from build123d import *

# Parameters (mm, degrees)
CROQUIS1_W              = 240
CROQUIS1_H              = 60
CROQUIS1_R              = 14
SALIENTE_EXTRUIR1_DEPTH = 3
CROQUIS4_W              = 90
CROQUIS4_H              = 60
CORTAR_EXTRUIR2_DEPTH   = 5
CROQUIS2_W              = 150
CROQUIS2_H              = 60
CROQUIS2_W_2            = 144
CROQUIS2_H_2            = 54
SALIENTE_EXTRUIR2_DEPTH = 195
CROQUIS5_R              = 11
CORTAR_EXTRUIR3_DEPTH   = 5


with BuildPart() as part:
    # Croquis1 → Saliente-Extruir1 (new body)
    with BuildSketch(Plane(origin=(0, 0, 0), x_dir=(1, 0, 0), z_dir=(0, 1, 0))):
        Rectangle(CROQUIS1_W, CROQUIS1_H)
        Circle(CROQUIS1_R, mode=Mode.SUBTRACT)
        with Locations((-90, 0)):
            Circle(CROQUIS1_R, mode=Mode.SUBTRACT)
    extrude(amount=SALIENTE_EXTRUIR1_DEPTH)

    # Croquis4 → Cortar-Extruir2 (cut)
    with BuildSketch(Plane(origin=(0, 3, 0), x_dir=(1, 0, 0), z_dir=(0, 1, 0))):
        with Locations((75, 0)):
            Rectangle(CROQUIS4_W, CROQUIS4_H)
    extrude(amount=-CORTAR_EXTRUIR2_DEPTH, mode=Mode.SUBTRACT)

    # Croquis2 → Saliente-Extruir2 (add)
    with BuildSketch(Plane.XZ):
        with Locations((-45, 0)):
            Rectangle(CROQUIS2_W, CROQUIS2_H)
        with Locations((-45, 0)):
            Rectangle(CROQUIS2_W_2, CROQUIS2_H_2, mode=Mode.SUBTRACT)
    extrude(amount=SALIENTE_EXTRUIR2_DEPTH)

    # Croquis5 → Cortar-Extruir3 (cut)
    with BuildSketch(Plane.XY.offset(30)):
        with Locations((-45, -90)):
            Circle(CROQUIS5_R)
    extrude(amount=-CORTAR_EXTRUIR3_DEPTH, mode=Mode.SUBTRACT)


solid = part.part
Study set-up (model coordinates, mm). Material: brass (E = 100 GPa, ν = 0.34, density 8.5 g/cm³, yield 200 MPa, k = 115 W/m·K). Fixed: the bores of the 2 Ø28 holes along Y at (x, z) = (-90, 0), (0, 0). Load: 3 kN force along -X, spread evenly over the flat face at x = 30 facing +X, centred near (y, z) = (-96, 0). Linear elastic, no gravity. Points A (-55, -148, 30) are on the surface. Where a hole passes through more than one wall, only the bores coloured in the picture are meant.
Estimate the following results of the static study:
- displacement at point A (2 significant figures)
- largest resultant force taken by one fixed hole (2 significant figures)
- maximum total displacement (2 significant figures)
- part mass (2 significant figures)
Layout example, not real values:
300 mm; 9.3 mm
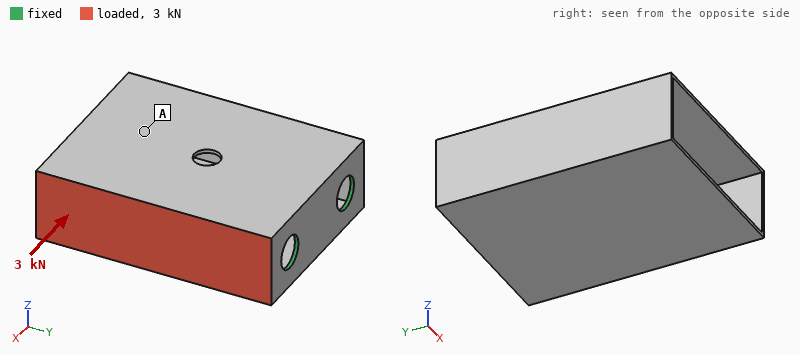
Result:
0.21 mm; 3.1 kN; 0.36 mm; 2.2 kg
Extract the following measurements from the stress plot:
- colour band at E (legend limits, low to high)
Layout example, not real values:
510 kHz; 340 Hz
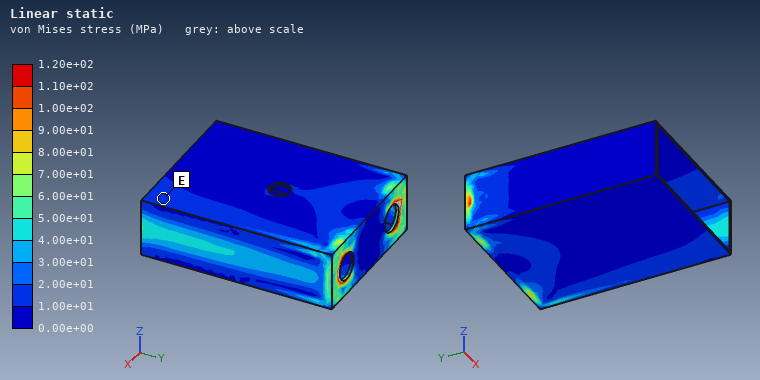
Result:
1.00e+01 to 2.00e+01 MPa
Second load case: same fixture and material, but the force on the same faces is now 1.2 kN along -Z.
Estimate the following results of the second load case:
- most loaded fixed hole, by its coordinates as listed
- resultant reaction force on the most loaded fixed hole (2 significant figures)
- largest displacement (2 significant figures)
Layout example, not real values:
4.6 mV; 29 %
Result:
(0, 0); 1.2 kN; 1.0 mm
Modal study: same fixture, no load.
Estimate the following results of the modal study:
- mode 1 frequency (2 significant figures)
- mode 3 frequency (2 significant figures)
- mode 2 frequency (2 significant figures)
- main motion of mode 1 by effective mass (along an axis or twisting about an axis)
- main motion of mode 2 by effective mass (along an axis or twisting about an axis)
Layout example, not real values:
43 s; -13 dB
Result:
170 Hz; 380 Hz; 300 Hz; along Z; twisting about Y
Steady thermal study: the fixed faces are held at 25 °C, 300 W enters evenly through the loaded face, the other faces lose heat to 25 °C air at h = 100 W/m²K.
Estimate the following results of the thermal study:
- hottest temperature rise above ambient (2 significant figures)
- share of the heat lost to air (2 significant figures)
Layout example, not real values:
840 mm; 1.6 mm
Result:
82 K; 86 %
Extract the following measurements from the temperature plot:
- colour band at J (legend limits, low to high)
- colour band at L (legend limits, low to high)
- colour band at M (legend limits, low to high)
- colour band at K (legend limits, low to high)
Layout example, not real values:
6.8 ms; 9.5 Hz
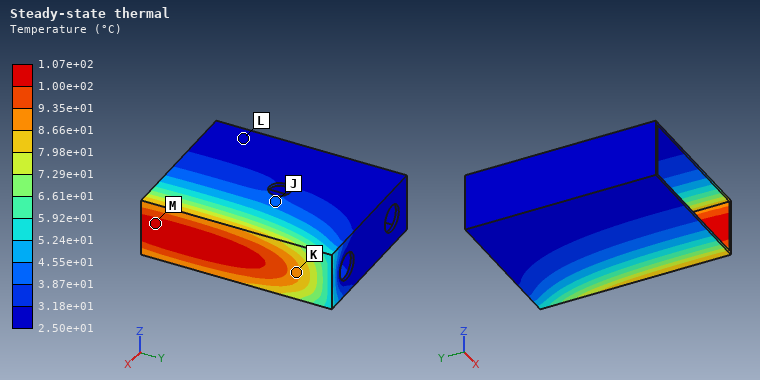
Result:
3.87e+01 to 4.55e+01 °C; 2.50e+01 to 3.18e+01 °C; 1.00e+02 to 1.07e+02 °C; 8.66e+01 to 9.35e+01 °C
